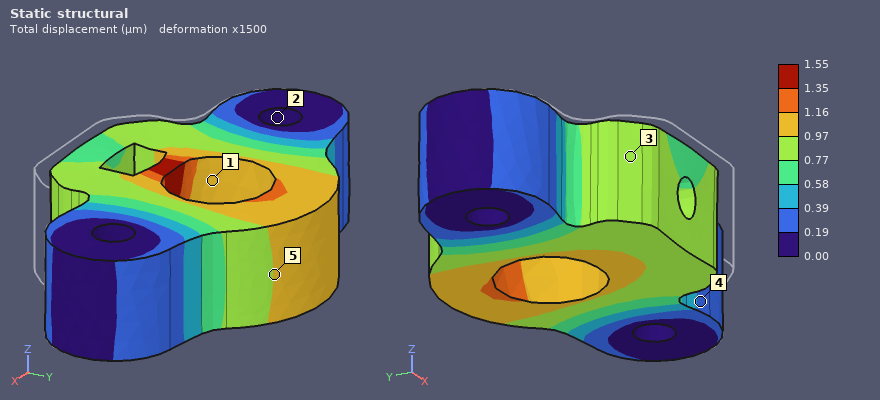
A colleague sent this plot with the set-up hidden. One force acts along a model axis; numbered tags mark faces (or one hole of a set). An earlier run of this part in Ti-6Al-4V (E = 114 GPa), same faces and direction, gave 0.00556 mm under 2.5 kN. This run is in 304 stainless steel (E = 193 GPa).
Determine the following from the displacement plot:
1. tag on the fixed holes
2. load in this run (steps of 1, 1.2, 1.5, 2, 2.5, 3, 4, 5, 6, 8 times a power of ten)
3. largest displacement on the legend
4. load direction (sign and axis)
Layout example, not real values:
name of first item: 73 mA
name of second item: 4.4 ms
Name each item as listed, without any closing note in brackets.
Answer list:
tag on the fixed holes: 2
load in this run: 1.2 kN
largest displacement on the legend: 1.55 µm
load direction: +Y
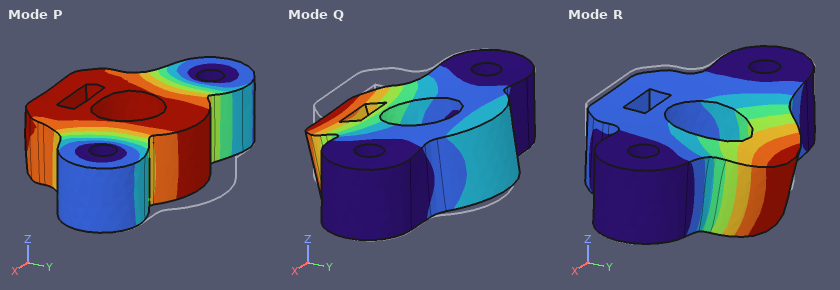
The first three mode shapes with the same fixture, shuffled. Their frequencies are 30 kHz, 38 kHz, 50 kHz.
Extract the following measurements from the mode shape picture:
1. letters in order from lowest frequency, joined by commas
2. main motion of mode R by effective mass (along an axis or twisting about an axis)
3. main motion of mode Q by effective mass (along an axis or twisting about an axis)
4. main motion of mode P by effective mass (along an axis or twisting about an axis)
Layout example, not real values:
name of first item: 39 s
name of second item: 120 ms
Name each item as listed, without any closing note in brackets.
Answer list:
letters in order from lowest frequency, joined by commas: Q, R, P
main motion of mode R by effective mass: along Z
main motion of mode Q by effective mass: along Z
main motion of mode P by effective mass: along Y
